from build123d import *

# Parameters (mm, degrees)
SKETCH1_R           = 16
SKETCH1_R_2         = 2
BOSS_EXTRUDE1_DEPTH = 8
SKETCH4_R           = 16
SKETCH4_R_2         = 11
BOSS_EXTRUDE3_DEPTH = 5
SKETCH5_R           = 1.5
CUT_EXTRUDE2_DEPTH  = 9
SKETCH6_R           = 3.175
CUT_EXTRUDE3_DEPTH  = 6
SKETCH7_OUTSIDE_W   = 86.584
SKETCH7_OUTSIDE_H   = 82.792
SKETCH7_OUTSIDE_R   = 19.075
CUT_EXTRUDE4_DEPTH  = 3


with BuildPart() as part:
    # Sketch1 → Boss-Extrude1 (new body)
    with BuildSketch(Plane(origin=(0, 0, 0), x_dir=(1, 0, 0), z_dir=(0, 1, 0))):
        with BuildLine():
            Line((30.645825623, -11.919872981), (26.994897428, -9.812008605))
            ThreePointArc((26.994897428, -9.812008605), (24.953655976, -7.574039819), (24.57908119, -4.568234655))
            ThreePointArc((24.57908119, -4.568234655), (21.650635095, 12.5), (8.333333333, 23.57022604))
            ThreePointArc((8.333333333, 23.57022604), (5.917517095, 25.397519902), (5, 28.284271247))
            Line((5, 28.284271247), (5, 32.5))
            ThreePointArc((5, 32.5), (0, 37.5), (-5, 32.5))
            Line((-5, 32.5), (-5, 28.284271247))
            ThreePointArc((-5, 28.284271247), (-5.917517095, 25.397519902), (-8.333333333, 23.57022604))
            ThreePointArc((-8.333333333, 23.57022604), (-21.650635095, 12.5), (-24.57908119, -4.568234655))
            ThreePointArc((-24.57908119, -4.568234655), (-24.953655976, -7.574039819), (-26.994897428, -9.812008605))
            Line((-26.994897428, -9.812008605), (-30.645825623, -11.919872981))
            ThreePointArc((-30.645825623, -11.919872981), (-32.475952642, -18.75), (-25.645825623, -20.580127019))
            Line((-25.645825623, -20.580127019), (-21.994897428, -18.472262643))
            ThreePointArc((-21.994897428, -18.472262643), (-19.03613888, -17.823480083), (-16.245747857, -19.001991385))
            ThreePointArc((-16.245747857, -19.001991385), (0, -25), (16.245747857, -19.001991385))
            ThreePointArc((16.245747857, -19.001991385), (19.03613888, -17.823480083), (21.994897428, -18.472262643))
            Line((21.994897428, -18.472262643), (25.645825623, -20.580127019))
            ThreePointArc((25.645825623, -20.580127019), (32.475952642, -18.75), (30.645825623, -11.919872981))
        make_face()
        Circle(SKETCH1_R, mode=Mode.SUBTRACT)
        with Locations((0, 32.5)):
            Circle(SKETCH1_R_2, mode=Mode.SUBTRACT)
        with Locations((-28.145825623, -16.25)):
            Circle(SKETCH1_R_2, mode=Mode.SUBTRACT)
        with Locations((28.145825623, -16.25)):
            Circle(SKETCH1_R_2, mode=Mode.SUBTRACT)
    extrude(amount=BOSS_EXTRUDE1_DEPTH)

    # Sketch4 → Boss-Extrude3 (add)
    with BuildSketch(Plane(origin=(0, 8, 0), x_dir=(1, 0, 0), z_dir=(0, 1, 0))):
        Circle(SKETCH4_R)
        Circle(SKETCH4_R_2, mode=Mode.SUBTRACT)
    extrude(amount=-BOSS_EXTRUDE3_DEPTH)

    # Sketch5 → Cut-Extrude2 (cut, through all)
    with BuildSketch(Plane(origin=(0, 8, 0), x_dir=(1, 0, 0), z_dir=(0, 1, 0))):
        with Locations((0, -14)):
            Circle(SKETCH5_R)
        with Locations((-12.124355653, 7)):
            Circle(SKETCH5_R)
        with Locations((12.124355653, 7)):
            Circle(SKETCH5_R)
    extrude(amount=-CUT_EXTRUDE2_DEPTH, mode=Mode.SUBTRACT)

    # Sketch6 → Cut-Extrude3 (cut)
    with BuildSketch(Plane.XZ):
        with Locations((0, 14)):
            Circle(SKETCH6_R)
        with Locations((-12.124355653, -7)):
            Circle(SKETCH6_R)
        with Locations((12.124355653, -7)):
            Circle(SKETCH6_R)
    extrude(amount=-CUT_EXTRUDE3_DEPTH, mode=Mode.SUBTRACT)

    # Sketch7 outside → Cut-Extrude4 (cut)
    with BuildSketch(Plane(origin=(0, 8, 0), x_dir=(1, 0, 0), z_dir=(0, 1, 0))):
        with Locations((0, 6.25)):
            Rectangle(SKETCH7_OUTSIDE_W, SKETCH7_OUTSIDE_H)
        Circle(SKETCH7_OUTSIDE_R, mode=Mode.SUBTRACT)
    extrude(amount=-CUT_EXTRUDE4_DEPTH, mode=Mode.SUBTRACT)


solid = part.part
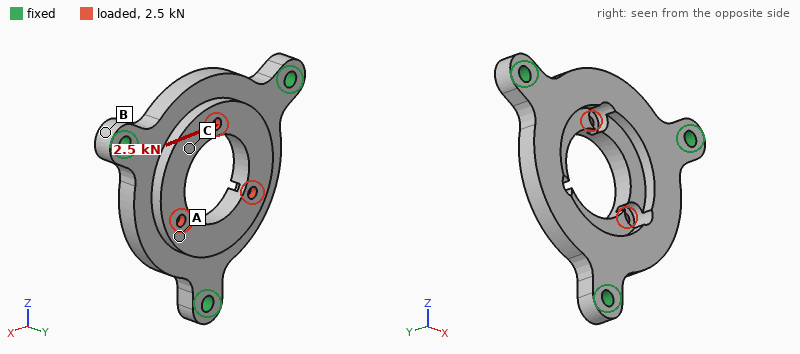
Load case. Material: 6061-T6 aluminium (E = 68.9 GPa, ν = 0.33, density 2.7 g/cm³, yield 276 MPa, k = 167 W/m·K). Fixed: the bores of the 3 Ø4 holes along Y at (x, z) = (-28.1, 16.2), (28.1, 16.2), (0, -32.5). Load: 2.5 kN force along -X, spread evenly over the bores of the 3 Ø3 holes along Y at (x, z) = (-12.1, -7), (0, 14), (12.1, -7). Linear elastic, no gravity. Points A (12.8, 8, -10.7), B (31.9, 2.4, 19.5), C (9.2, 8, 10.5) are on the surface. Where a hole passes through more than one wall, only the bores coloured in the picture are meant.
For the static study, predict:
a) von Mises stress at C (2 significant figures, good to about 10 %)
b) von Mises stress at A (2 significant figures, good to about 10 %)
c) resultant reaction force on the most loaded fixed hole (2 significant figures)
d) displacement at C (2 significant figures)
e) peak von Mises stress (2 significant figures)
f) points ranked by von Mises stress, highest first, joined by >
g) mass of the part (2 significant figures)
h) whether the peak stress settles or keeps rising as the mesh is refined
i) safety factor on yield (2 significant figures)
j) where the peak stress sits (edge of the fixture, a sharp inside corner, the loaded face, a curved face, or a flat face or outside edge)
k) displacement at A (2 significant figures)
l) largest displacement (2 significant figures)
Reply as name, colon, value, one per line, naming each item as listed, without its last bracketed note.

von Mises stress at C: 18 MPa
von Mises stress at A: 28 MPa
resultant reaction force on the most loaded fixed hole: 910 N
displacement at C: 9.9 µm
peak von Mises stress: 140 MPa
points ranked by von Mises stress, highest first, joined by >: A > C > B
mass of the part: 28 g
whether the peak stress settles or keeps rising as the mesh is refined: settles
safety factor on yield: 1.9
where the peak stress sits: a curved face
displacement at A: 26 µm
largest displacement: 29 µm
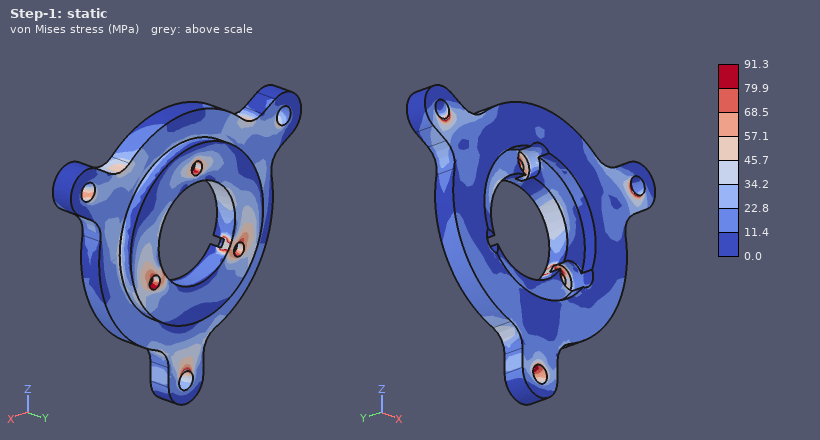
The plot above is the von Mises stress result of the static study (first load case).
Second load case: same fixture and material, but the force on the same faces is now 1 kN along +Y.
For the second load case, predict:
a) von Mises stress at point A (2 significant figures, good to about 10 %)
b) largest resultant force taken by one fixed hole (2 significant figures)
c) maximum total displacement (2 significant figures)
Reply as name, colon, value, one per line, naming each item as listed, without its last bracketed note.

von Mises stress at point A: 43 MPa
largest resultant force taken by one fixed hole: 520 N
maximum total displacement: 37 µm
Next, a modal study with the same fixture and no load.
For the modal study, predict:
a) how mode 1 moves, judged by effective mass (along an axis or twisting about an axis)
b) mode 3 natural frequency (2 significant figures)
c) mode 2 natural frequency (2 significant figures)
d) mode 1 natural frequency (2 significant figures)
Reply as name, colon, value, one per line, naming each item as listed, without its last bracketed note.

how mode 1 moves, judged by effective mass: along Y
mode 3 natural frequency: 8000 Hz
mode 2 natural frequency: 8000 Hz
mode 1 natural frequency: 7400 Hz
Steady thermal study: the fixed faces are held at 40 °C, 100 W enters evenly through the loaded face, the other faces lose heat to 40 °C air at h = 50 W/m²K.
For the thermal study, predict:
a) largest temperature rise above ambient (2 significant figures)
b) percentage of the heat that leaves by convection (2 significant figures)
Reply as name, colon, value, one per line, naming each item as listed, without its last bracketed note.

largest temperature rise above ambient: 78 K
percentage of the heat that leaves by convection: 11 %
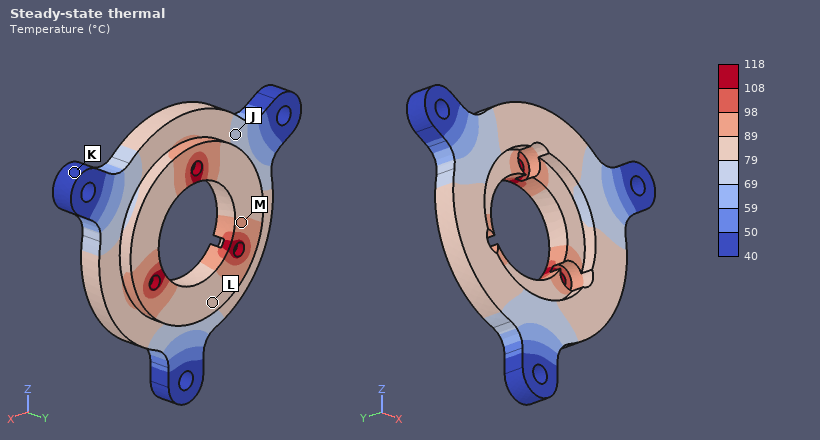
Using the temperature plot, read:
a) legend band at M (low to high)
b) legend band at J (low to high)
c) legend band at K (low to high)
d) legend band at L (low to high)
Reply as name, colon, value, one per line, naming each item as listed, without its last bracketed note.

legend band at M: 89 to 98 °C
legend band at J: 69 to 79 °C
legend band at K: 40 to 50 °C
legend band at L: 79 to 89 °C
